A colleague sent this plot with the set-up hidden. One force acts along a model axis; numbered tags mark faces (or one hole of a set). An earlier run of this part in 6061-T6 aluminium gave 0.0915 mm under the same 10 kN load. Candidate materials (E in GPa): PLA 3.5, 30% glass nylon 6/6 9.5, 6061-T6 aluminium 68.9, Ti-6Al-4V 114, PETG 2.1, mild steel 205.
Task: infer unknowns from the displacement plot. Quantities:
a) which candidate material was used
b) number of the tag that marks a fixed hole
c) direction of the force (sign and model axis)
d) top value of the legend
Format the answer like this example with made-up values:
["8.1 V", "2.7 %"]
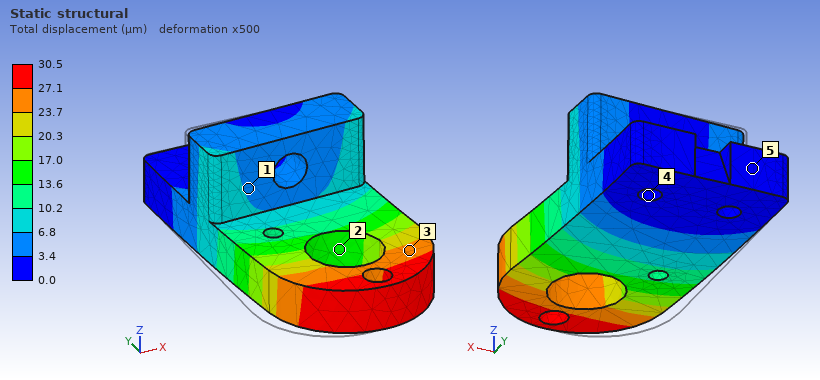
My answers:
["mild steel", "4", "+X", "30.5 µm"]
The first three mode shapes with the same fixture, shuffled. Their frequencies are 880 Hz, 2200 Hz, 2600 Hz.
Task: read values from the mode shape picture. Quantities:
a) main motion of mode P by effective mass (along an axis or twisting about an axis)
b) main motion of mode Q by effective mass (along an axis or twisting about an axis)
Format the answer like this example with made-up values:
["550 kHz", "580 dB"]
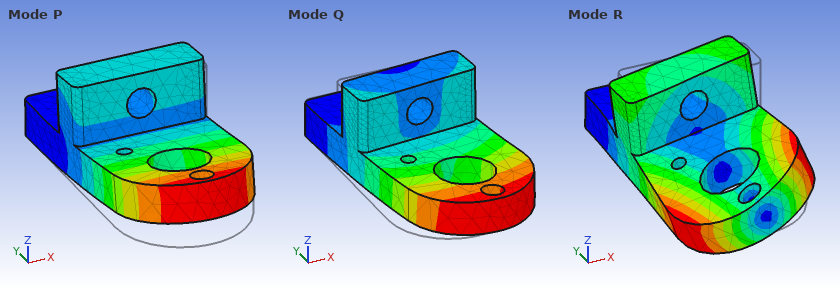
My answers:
["along Z", "along X"]
